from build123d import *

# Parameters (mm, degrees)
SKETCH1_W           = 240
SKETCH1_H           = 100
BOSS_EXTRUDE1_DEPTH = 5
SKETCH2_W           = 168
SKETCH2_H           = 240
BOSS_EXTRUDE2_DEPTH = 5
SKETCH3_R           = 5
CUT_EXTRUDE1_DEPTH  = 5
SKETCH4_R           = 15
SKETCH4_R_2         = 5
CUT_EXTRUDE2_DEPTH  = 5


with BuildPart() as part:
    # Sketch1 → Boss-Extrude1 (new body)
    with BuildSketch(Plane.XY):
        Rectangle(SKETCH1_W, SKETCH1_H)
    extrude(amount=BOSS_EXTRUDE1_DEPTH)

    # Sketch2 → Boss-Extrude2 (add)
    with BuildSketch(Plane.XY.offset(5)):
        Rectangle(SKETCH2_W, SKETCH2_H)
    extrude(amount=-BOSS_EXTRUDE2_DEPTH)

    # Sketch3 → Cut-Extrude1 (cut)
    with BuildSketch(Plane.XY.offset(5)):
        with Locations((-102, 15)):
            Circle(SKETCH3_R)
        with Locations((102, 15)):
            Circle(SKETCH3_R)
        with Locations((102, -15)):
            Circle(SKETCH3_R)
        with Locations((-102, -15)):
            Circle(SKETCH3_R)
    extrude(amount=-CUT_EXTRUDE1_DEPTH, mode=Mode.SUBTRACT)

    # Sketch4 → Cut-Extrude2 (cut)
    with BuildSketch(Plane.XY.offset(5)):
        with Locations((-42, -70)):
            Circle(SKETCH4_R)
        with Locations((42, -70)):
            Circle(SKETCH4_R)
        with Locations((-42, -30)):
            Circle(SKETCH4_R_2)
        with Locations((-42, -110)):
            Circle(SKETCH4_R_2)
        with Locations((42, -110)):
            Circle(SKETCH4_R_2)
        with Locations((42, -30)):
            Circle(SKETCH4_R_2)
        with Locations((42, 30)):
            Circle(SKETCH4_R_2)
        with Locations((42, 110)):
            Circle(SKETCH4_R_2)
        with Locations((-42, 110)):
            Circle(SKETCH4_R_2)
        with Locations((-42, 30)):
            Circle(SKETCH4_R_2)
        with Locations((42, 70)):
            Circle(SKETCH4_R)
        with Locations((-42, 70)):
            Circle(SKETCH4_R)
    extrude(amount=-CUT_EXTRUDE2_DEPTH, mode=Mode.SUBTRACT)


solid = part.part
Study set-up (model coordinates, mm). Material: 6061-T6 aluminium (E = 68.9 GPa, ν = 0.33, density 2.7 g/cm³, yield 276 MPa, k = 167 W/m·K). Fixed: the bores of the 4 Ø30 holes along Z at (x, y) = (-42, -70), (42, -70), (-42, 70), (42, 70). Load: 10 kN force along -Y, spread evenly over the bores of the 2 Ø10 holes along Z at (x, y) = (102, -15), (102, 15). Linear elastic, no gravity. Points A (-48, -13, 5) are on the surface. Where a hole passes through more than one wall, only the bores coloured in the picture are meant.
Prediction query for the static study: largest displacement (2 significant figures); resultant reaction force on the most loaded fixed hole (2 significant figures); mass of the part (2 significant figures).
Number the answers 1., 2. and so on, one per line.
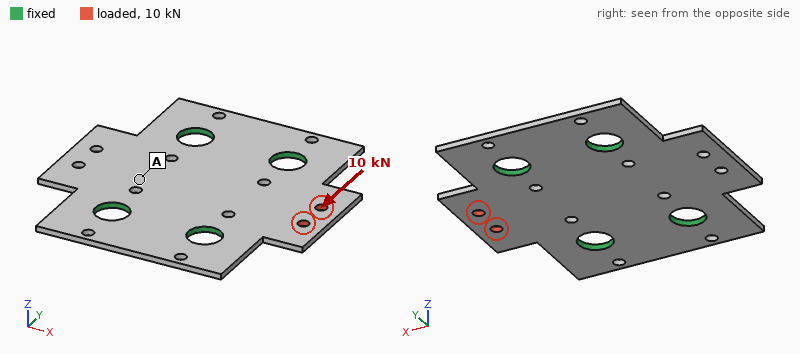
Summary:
1. 53 µm
2. 6.1 kN
3. 590 g
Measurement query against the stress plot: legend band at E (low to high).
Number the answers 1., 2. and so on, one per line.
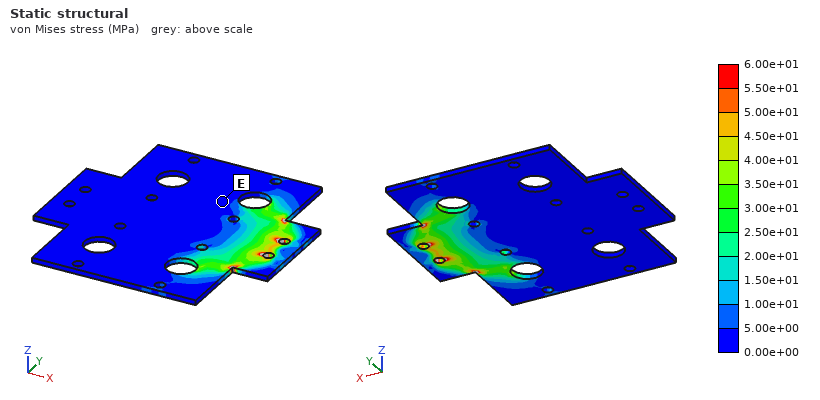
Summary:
1. 0.00e+00 to 5.00e+00 MPa
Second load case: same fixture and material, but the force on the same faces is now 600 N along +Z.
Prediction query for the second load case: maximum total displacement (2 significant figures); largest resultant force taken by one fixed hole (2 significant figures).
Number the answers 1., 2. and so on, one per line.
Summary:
1. 0.74 mm
2. 340 N
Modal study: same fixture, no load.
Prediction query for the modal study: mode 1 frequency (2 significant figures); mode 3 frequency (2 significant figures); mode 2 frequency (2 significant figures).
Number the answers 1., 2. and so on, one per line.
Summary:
1. 790 Hz
2. 1900 Hz
3. 790 Hz
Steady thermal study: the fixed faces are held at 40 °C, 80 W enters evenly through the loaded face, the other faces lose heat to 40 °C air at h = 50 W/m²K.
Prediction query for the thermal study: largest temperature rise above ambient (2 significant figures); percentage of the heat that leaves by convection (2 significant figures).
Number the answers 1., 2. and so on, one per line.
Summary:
1. 55 K
2. 35 %
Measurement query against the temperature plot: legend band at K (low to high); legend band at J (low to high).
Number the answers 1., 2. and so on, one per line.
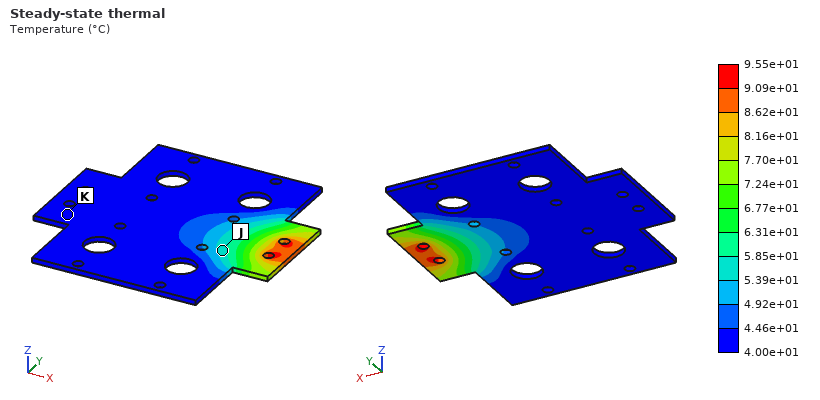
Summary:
1. 4.00e+01 to 4.46e+01 °C
2. 5.39e+01 to 5.85e+01 °C
